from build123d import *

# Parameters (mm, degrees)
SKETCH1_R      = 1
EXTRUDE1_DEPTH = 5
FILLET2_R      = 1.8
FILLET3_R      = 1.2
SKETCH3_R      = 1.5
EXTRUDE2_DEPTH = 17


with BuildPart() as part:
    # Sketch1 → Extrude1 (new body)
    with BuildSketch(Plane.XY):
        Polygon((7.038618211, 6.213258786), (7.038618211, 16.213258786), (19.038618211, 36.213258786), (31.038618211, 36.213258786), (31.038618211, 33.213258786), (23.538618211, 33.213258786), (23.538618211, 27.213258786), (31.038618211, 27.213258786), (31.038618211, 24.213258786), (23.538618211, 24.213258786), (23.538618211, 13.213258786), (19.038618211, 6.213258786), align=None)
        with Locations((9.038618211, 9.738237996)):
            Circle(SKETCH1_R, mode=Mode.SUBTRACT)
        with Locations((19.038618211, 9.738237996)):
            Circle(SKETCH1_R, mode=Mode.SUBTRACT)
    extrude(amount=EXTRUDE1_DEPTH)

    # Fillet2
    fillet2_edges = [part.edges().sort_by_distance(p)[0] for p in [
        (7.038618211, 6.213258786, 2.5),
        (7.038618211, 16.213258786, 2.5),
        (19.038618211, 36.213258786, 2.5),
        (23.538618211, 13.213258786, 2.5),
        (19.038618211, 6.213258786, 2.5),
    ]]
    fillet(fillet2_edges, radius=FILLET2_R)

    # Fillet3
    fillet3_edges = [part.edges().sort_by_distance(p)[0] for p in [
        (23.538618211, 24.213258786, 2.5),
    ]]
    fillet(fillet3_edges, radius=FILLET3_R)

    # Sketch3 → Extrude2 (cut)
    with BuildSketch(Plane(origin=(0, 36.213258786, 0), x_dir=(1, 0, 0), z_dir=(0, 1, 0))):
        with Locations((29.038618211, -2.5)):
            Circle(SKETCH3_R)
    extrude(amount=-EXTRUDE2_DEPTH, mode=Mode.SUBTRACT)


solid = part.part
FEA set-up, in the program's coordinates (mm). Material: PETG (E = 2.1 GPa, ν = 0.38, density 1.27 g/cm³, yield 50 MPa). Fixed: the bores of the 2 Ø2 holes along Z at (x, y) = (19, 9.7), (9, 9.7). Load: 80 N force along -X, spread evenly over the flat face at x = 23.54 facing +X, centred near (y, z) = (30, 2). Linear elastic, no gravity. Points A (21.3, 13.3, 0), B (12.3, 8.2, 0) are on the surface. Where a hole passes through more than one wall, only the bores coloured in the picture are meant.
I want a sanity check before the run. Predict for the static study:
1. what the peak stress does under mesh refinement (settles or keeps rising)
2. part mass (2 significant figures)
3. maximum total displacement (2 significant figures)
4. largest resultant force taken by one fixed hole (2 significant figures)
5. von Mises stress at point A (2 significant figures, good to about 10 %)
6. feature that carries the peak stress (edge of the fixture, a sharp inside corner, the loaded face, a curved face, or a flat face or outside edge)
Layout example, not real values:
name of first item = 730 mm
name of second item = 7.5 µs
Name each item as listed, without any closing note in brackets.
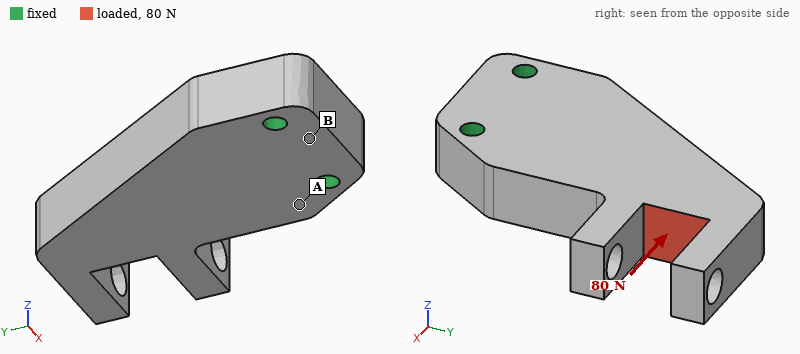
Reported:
what the peak stress does under mesh refinement = keeps rising
part mass = 2.5 g
maximum total displacement = 0.21 mm
largest resultant force taken by one fixed hole = 160 N
von Mises stress at point A = 5.0 MPa
feature that carries the peak stress = edge of the fixture
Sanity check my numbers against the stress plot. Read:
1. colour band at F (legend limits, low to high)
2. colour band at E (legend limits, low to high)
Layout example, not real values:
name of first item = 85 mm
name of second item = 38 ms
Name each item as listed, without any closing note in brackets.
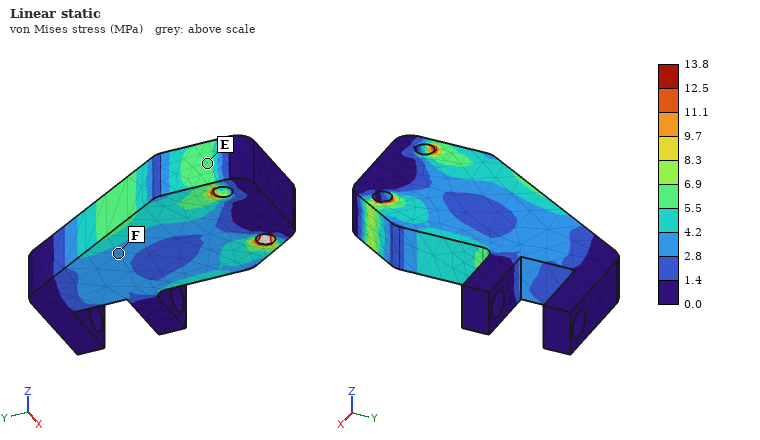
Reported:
colour band at F = 2.8 to 4.2 MPa
colour band at E = 5.5 to 6.9 MPa
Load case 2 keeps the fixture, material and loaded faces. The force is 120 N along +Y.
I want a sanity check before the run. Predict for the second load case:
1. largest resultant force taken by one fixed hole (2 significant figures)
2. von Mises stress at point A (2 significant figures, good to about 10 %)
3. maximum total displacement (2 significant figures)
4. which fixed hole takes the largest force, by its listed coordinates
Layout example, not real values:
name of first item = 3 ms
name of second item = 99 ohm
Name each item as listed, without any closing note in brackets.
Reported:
largest resultant force taken by one fixed hole = 170 N
von Mises stress at point A = 5.7 MPa
maximum total displacement = 0.23 mm
which fixed hole takes the largest force, by its listed coordinates = (19, 9.7)
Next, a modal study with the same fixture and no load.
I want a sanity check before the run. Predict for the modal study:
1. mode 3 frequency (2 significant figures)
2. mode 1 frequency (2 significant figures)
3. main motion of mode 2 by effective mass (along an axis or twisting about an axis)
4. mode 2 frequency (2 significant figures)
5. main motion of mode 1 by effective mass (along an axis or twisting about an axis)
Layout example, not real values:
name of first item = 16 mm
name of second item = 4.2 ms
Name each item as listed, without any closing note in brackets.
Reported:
mode 3 frequency = 4900 Hz
mode 1 frequency = 1500 Hz
main motion of mode 2 by effective mass = along X
mode 2 frequency = 3700 Hz
main motion of mode 1 by effective mass = along Z
